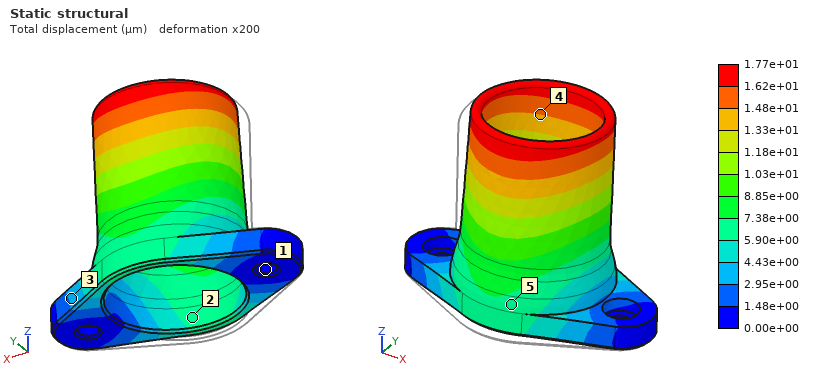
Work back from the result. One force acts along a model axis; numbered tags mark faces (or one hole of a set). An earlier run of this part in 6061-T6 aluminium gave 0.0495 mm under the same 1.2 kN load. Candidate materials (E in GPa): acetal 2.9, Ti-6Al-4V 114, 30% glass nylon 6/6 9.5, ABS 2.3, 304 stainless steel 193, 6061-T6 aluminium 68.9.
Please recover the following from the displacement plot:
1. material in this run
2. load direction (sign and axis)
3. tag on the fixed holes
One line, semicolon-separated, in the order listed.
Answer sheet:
304 stainless steel; +Y; 1
